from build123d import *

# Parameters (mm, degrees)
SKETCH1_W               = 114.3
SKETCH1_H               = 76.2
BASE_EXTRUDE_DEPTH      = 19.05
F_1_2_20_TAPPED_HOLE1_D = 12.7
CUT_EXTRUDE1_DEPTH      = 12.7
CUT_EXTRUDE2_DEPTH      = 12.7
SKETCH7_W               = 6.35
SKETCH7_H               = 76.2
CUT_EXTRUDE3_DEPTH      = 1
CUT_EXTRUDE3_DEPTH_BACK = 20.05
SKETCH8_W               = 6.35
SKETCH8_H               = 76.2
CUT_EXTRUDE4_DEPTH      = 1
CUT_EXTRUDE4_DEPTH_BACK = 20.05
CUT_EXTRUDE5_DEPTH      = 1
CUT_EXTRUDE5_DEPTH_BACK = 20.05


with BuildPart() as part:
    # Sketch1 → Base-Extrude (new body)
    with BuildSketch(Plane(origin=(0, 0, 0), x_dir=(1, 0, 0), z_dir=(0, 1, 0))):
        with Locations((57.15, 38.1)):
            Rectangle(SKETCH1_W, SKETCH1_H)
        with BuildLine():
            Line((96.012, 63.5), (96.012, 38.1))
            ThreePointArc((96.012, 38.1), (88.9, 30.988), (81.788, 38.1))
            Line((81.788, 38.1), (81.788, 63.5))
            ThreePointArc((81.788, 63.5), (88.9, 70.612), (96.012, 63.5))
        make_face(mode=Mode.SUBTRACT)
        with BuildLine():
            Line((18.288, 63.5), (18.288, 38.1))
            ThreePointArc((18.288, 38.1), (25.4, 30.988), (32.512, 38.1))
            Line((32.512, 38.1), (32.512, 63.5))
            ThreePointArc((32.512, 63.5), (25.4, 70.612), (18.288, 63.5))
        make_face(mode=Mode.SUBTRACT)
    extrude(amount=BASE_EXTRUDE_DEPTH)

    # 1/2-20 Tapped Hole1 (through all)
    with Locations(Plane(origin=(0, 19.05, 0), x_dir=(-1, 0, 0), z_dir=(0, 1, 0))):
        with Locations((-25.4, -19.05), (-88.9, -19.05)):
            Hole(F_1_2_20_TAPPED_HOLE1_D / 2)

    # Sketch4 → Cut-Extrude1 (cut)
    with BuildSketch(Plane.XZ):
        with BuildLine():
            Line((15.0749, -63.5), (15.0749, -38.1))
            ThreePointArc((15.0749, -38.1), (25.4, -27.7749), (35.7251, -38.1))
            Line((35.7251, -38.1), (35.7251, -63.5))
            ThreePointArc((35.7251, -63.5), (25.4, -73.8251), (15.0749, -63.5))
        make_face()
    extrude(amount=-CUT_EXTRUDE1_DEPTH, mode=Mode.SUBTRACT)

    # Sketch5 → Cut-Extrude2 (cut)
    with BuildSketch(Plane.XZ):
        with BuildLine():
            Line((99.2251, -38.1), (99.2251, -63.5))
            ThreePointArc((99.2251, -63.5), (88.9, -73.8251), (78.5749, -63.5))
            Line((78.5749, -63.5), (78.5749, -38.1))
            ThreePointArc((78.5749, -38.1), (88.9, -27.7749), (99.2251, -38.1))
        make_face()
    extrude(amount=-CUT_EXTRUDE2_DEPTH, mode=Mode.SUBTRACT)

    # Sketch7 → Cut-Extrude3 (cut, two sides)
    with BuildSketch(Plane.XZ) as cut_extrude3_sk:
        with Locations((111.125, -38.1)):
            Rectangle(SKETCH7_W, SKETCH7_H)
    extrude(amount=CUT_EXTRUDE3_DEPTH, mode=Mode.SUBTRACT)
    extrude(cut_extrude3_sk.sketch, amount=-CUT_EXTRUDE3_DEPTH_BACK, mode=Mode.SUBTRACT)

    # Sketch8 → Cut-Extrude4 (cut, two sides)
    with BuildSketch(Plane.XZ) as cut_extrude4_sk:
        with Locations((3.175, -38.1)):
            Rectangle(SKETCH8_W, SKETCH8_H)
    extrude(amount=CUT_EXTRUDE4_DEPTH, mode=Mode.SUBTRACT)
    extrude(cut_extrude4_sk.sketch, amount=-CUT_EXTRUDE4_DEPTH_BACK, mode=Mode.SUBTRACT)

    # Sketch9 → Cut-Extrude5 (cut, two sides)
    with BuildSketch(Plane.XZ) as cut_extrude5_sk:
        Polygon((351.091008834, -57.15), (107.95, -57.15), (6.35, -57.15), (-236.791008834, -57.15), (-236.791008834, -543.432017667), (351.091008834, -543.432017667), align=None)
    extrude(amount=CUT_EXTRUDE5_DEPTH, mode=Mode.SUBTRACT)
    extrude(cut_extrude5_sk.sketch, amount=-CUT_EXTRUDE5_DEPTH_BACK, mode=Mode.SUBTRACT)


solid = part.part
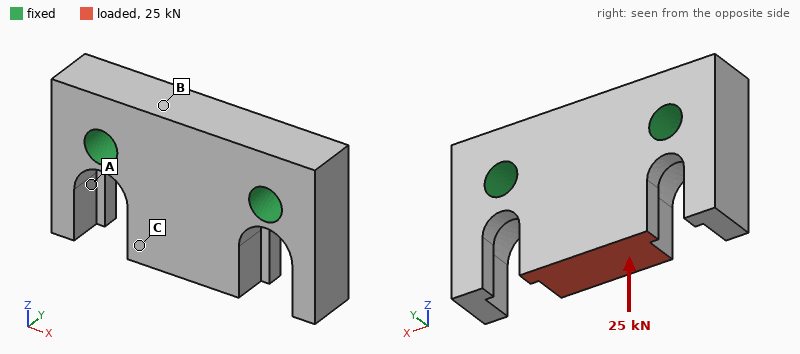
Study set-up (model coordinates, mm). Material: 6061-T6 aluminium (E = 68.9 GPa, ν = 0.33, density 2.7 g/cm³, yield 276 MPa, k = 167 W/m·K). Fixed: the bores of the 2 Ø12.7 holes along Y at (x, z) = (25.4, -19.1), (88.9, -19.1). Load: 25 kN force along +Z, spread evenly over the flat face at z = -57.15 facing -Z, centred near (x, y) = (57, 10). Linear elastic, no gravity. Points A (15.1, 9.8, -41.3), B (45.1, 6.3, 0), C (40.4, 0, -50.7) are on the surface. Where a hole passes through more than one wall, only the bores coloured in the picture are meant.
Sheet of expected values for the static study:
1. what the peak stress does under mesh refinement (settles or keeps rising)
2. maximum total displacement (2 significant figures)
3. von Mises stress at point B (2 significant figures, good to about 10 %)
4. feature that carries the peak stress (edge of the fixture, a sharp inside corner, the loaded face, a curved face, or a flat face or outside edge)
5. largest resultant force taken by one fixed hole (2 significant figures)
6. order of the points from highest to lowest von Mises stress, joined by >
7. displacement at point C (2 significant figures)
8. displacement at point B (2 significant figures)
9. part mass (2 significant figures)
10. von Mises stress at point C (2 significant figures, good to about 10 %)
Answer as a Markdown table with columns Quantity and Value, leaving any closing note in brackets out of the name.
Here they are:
| Quantity | Value |
|---|---|
| what the peak stress does under mesh refinement | keeps rising |
| maximum total displacement | 26 µm |
| von Mises stress at point B | 18 MPa |
| feature that carries the peak stress | edge of the fixture |
| largest resultant force taken by one fixed hole | 13 kN |
| order of the points from highest to lowest von Mises stress, joined by > | C > B > A |
| displacement at point C | 22 µm |
| displacement at point B | 11 µm |
| part mass | 240 g |
| von Mises stress at point C | 31 MPa |
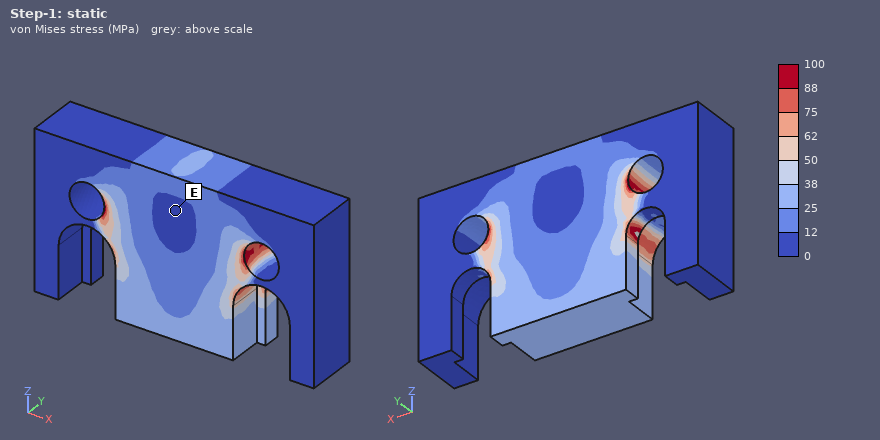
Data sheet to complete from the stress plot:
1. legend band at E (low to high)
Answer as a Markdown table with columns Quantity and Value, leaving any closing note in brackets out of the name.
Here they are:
| Quantity | Value |
|---|---|
| legend band at E | 0 to 12 MPa |
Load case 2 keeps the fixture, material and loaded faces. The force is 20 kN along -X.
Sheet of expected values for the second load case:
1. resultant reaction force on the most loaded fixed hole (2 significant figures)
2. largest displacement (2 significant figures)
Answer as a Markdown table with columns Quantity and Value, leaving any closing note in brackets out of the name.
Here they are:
| Quantity | Value |
|---|---|
| resultant reaction force on the most loaded fixed hole | 16 kN |
| largest displacement | 69 µm |
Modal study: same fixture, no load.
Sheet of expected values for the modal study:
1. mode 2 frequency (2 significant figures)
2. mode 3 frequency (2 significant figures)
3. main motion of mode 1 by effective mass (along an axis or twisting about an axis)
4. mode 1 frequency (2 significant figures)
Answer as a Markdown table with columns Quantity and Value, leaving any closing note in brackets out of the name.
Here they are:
| Quantity | Value |
|---|---|
| mode 2 frequency | 8400 Hz |
| mode 3 frequency | 8400 Hz |
| main motion of mode 1 by effective mass | along Y |
| mode 1 frequency | 7500 Hz |
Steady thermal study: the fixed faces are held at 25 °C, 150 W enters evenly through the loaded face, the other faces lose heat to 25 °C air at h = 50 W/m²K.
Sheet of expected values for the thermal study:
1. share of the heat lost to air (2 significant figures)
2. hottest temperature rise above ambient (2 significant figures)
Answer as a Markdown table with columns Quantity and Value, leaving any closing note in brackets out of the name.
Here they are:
| Quantity | Value |
|---|---|
| share of the heat lost to air | 4.6 % |
| hottest temperature rise above ambient | 43 K |
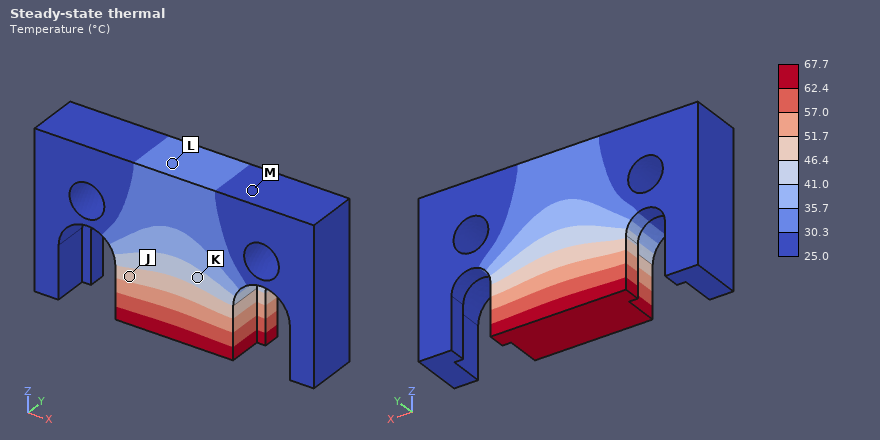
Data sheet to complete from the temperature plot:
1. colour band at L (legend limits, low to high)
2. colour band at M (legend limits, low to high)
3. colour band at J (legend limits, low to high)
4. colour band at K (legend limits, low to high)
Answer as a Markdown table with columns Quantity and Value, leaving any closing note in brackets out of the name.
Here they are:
| Quantity | Value |
|---|---|
| colour band at L | 30.3 to 35.7 °C |
| colour band at M | 25.0 to 30.3 °C |
| colour band at J | 46.4 to 51.7 °C |
| colour band at K | 41.0 to 46.4 °C |
